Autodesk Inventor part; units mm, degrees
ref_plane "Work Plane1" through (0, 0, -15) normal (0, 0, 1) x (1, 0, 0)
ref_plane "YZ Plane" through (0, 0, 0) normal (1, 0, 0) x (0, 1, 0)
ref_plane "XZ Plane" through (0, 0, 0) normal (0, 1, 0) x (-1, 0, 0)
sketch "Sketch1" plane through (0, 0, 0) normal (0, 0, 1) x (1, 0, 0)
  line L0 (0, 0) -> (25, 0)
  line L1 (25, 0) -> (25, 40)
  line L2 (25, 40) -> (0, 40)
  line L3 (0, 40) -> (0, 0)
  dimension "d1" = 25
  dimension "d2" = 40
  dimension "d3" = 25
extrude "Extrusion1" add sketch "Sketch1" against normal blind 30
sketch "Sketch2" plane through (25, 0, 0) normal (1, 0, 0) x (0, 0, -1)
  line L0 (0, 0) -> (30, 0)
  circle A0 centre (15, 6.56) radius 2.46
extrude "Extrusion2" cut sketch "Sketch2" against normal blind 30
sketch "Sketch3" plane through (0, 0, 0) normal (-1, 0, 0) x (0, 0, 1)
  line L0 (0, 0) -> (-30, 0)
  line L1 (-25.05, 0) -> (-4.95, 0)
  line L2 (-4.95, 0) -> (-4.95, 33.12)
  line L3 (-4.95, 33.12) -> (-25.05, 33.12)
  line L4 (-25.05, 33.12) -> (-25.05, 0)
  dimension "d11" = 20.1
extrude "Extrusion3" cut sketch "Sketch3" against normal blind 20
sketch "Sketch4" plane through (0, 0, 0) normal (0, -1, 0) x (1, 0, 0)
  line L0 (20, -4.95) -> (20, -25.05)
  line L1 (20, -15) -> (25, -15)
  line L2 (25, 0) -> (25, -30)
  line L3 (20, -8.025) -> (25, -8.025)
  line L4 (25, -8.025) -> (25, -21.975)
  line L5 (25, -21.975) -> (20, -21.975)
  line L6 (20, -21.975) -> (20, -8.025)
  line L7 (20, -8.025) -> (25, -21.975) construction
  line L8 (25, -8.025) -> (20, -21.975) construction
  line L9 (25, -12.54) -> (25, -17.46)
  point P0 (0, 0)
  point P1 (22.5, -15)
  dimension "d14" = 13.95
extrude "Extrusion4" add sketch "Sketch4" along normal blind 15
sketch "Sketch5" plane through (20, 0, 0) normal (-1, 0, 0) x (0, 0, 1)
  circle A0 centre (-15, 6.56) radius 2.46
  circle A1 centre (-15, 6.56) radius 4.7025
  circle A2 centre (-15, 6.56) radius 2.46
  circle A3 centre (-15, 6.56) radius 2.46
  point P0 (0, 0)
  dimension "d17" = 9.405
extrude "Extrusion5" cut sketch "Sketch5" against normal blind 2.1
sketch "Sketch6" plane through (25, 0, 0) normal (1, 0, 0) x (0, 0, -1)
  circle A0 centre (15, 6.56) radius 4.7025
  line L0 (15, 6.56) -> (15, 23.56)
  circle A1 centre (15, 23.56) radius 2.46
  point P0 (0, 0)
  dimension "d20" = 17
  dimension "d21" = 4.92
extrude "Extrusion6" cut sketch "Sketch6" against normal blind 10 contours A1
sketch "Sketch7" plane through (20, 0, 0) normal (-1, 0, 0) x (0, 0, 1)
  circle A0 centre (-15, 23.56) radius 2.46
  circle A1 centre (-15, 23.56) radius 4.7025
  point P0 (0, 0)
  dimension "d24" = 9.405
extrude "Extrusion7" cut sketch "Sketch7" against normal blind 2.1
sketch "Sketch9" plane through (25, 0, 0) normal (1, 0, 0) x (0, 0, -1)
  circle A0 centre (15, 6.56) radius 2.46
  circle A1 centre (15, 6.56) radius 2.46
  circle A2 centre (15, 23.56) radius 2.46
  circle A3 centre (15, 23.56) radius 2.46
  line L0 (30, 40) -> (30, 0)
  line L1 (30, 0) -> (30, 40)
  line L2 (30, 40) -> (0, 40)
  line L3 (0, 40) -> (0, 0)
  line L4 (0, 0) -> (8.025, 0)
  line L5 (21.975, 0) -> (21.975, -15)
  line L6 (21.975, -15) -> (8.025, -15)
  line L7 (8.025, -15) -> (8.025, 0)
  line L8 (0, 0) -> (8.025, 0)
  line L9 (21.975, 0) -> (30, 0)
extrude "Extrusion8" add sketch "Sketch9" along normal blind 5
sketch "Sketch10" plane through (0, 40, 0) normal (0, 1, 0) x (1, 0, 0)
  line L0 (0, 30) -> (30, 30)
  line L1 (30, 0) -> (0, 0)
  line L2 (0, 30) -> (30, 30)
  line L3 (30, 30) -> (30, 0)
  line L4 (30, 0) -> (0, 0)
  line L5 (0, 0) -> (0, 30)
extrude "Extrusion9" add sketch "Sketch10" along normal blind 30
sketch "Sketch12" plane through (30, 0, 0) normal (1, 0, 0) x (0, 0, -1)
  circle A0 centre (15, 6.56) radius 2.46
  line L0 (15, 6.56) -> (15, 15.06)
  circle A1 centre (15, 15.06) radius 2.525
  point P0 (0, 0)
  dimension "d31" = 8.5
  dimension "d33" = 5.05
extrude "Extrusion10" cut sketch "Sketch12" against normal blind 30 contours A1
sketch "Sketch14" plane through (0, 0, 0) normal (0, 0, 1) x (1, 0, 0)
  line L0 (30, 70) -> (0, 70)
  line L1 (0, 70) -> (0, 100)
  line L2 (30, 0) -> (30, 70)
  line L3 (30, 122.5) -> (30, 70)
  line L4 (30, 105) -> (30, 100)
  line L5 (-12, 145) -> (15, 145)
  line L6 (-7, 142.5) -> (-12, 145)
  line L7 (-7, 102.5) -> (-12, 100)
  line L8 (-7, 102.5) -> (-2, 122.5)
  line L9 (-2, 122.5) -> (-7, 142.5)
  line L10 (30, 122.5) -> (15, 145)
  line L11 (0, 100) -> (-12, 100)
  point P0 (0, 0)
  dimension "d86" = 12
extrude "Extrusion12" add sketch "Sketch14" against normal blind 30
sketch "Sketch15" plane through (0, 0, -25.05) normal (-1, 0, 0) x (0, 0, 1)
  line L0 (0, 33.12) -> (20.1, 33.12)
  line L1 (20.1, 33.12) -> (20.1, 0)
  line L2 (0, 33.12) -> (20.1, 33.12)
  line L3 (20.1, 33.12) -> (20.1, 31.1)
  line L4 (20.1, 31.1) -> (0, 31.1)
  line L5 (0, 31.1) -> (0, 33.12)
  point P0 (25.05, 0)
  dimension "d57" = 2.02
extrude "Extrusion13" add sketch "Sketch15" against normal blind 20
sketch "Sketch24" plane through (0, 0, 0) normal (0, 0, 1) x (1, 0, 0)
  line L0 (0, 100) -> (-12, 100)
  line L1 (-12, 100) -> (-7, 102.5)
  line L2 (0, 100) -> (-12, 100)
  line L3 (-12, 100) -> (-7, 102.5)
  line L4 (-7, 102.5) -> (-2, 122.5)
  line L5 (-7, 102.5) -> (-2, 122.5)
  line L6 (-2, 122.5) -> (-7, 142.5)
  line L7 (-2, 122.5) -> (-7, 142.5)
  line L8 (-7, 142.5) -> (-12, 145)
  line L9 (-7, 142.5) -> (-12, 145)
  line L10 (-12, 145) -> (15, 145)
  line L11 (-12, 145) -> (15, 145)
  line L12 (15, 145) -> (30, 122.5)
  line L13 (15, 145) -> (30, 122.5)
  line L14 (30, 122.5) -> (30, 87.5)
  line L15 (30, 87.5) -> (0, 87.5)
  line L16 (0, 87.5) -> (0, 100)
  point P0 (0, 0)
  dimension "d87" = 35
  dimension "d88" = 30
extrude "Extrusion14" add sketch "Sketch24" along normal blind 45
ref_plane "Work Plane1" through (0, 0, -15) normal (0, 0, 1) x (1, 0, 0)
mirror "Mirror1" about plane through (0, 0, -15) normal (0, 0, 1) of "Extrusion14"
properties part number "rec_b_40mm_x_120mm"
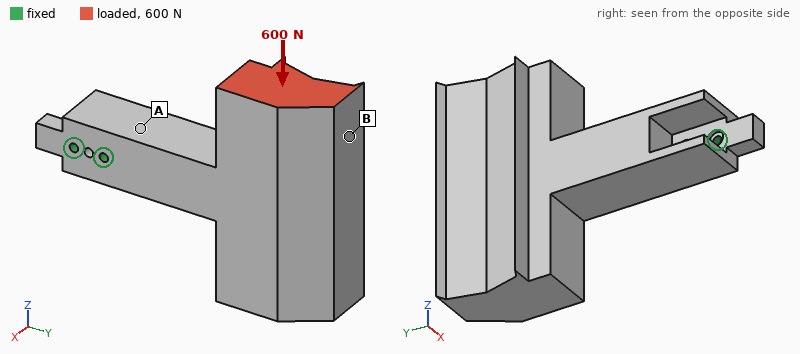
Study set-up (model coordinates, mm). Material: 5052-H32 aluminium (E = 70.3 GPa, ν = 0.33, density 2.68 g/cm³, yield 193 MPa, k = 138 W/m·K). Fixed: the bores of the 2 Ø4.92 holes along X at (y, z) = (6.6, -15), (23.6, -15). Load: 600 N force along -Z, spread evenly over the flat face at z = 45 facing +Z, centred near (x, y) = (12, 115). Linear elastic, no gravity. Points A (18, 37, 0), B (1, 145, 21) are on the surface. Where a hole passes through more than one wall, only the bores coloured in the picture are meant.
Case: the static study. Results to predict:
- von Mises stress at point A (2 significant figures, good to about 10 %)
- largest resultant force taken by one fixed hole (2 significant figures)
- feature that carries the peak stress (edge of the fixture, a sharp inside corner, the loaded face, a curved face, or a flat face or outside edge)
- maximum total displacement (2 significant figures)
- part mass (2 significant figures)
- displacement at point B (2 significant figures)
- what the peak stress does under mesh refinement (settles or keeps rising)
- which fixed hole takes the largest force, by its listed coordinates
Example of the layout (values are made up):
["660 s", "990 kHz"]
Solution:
["14 MPa", "3.0 kN", "edge of the fixture", "0.16 mm", "750 g", "0.15 mm", "keeps rising", "(23.6, -15)"]
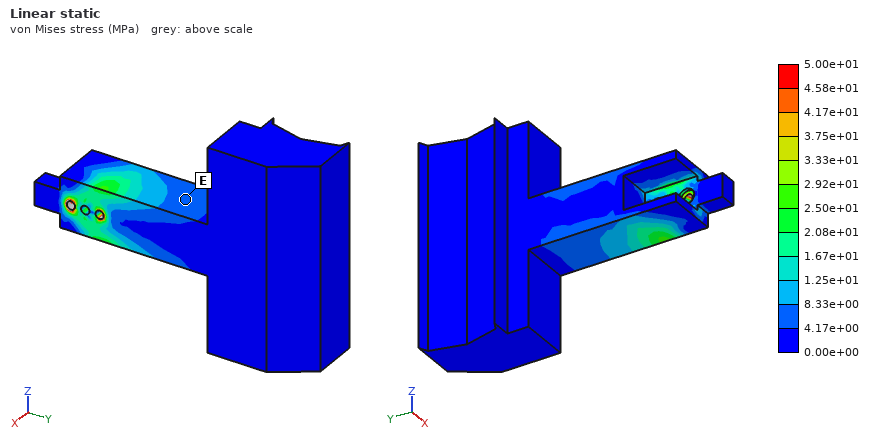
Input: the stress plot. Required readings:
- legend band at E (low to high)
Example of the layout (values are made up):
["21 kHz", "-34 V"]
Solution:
["4.17e+00 to 8.33e+00 MPa"]
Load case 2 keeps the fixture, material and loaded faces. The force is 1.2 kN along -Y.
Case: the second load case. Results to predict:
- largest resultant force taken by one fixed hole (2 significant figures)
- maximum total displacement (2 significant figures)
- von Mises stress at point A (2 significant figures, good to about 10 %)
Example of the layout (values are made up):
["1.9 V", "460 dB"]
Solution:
["3.3 kN", "0.27 mm", "26 MPa"]
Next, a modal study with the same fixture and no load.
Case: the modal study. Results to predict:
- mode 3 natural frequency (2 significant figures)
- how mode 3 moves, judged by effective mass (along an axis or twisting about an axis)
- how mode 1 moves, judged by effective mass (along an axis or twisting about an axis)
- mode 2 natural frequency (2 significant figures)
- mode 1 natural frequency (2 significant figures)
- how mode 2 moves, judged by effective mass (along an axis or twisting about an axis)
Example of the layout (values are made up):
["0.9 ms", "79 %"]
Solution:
["700 Hz", "twisting about Y", "along X", "450 Hz", "420 Hz", "along Z"]
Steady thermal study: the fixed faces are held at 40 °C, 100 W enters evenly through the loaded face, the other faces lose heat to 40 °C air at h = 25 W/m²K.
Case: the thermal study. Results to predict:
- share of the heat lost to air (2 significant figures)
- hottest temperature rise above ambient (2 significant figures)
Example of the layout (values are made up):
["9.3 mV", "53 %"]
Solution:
["40 %", "72 K"]
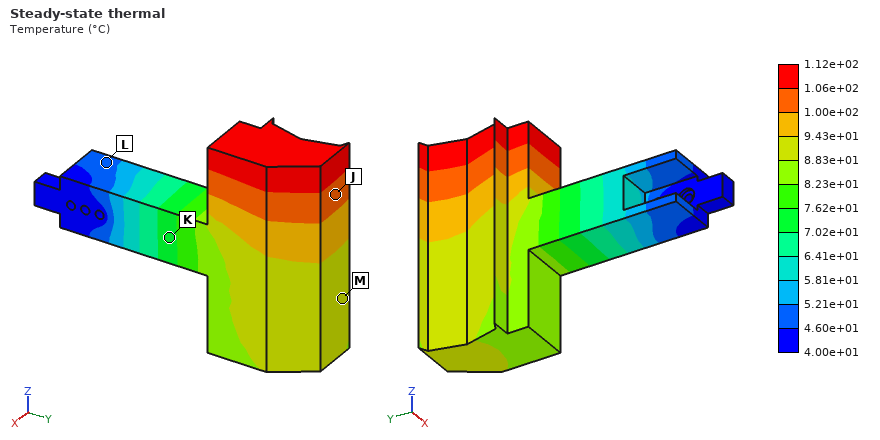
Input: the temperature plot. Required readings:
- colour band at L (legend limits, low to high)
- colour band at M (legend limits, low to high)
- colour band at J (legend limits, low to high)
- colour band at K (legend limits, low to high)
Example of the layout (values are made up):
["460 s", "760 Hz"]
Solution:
["4.60e+01 to 5.21e+01 °C", "8.83e+01 to 9.43e+01 °C", "1.00e+02 to 1.06e+02 °C", "7.02e+01 to 7.62e+01 °C"]
